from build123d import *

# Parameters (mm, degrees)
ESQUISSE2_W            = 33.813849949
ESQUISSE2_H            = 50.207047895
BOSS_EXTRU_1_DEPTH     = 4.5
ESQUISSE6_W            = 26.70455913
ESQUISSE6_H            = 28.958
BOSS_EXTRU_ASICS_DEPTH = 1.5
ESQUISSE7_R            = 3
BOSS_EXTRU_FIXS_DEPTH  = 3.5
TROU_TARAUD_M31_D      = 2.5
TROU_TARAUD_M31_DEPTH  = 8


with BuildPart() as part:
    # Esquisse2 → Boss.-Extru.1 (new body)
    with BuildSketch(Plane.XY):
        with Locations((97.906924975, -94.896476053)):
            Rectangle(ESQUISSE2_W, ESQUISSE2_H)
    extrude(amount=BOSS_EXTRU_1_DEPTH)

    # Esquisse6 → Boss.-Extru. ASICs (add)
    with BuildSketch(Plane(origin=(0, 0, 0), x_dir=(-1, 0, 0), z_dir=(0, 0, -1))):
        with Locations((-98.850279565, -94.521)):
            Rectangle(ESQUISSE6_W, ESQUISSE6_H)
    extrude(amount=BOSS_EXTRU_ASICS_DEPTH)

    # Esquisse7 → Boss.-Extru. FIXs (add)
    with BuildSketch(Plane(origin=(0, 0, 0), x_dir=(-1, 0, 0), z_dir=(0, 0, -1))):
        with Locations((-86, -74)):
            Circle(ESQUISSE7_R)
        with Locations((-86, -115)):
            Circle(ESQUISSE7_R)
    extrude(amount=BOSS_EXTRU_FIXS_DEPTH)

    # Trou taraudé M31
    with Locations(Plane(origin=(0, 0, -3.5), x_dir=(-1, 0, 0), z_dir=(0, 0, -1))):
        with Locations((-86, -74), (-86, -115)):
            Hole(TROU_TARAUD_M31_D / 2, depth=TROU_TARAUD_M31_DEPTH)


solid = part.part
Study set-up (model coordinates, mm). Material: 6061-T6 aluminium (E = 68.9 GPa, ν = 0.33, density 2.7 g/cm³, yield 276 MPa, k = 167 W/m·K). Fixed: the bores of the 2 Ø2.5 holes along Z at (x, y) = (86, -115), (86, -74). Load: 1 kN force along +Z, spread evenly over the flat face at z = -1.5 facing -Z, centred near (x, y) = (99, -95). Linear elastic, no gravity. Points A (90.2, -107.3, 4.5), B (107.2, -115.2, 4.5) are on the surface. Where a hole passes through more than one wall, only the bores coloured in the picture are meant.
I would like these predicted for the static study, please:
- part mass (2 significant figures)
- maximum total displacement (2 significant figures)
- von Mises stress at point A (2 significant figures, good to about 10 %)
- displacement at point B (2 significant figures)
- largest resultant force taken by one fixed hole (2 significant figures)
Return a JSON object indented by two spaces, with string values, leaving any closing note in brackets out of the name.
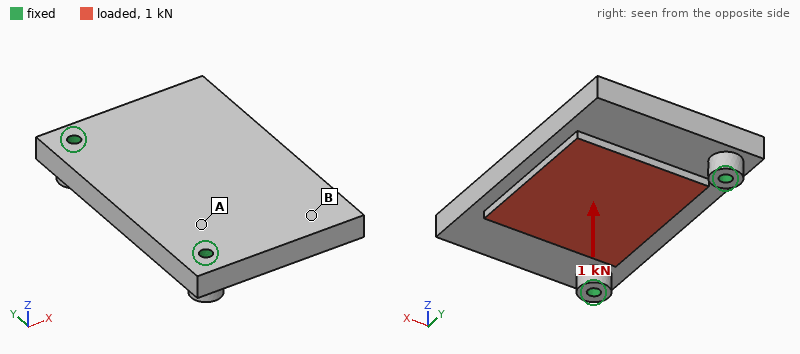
{
  "part mass": "24 g",
  "maximum total displacement": "0.16 mm",
  "von Mises stress at point A": "40 MPa",
  "displacement at point B": "0.094 mm",
  "largest resultant force taken by one fixed hole": "510 N"
}
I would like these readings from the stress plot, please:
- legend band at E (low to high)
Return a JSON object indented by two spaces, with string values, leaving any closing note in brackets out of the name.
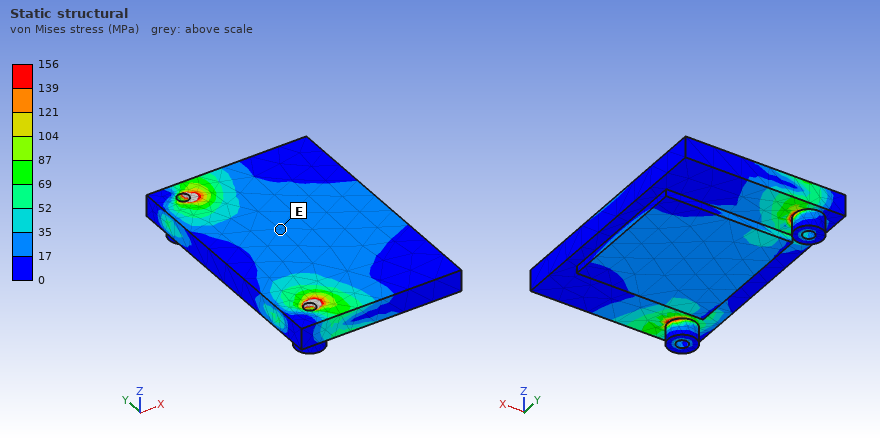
{
  "legend band at E": "17 to 35 MPa"
}
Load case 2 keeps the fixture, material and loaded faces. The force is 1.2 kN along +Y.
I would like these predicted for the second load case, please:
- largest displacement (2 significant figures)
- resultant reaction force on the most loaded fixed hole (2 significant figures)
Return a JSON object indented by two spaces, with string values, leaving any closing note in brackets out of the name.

{
  "largest displacement": "11 µm",
  "resultant reaction force on the most loaded fixed hole": "720 N"
}
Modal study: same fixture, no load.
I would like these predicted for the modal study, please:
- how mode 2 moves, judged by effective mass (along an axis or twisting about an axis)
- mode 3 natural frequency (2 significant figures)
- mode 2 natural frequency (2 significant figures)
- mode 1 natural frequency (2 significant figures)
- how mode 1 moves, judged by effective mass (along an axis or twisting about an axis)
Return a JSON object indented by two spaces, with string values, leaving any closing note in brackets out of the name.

{
  "how mode 2 moves, judged by effective mass": "twisting about X",
  "mode 3 natural frequency": "13 kHz",
  "mode 2 natural frequency": "8300 Hz",
  "mode 1 natural frequency": "3400 Hz",
  "how mode 1 moves, judged by effective mass": "along Z"
}
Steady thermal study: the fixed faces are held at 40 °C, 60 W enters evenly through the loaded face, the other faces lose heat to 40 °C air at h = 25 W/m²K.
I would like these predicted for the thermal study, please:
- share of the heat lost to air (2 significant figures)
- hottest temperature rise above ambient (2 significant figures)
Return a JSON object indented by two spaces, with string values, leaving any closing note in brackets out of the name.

{
  "share of the heat lost to air": "3.4 %",
  "hottest temperature rise above ambient": "36 K"
}
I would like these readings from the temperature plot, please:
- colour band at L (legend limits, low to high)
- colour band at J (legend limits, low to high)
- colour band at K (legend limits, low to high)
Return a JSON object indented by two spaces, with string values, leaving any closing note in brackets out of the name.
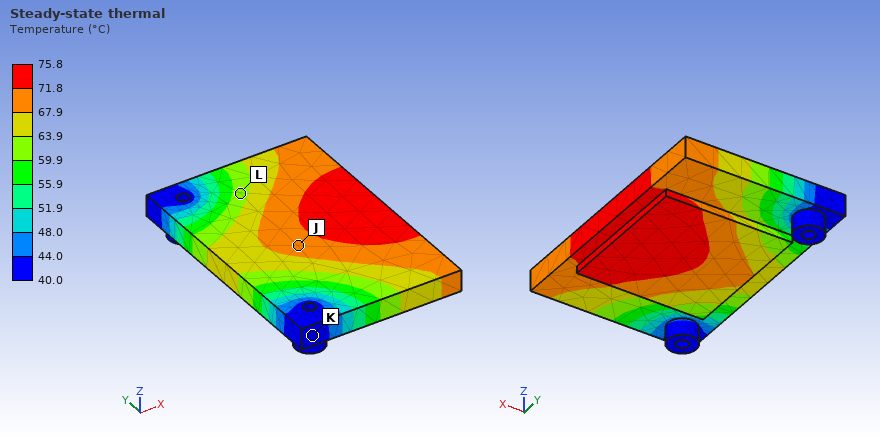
{
  "colour band at L": "59.9 to 63.9 °C",
  "colour band at J": "67.9 to 71.8 °C",
  "colour band at K": "40.0 to 44.0 °C"
}
